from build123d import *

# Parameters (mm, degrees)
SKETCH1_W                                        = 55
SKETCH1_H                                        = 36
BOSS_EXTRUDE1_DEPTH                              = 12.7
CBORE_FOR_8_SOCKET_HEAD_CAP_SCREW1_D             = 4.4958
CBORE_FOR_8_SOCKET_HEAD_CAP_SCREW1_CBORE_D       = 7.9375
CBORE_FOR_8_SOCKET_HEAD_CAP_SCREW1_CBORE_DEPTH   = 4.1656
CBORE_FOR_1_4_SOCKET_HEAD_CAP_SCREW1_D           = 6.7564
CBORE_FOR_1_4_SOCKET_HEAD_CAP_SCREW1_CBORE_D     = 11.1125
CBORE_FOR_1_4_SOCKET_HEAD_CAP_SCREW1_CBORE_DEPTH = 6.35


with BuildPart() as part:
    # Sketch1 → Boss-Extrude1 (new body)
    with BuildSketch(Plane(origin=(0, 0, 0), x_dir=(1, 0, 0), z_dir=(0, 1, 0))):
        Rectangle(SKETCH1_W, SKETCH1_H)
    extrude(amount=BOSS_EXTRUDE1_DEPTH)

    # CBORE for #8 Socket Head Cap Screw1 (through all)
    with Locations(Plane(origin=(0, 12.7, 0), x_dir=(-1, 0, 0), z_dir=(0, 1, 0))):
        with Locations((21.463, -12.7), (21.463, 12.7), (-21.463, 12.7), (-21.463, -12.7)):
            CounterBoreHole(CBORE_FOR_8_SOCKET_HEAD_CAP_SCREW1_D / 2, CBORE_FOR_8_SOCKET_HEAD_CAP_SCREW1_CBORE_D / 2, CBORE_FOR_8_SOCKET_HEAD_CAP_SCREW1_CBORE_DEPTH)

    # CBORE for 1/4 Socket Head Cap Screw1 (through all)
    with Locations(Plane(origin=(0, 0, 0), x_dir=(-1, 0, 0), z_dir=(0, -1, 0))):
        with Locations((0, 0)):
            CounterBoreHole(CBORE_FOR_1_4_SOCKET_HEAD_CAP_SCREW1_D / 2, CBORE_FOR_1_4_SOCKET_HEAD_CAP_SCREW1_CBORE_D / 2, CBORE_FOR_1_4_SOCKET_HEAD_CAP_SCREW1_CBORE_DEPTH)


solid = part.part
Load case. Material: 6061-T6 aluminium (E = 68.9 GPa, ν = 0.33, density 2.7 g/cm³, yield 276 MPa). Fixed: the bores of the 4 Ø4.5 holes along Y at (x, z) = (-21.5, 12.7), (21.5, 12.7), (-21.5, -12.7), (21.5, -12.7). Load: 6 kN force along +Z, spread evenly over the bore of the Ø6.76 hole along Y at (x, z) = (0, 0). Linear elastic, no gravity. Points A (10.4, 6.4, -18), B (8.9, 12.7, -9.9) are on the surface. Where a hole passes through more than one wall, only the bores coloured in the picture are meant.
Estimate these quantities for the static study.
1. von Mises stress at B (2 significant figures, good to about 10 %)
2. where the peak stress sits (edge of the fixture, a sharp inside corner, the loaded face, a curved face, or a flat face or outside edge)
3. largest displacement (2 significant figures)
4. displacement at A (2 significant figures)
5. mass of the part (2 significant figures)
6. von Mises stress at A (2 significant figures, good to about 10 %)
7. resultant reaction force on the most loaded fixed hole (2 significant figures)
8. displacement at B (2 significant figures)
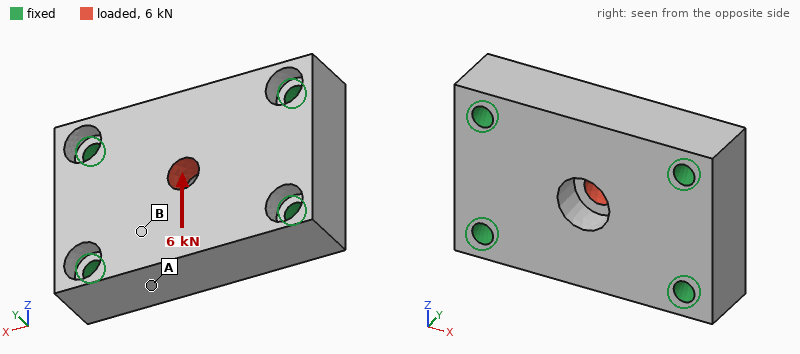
21 MPa
the loaded face
12 µm
5.0 µm
62 g
7.7 MPa
1.9 kN
6.0 µm
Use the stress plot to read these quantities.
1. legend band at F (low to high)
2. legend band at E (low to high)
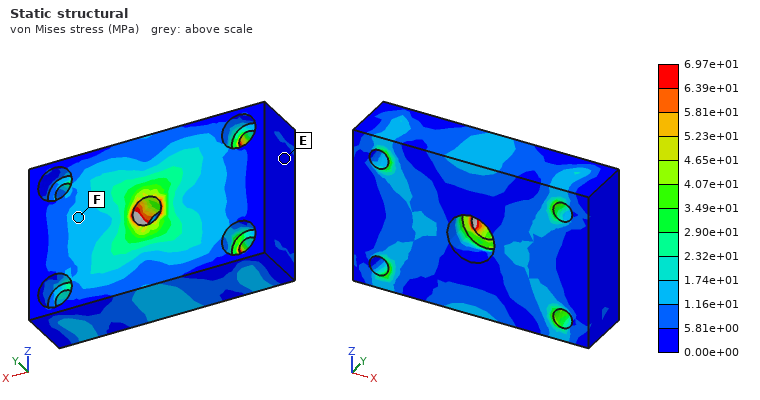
1.16e+01 to 1.74e+01 MPa
0.00e+00 to 5.81e+00 MPa
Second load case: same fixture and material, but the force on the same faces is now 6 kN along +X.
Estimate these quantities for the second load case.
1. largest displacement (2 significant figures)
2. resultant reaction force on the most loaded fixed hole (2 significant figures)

7.6 µm
1.6 kN
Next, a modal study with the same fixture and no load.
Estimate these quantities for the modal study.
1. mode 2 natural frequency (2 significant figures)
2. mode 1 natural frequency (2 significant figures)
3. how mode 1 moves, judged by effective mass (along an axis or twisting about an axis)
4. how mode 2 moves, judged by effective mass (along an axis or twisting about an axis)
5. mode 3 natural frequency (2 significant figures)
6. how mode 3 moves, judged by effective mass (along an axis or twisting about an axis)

26 kHz
20 kHz
along Y
twisting about X
30 kHz
along Z
